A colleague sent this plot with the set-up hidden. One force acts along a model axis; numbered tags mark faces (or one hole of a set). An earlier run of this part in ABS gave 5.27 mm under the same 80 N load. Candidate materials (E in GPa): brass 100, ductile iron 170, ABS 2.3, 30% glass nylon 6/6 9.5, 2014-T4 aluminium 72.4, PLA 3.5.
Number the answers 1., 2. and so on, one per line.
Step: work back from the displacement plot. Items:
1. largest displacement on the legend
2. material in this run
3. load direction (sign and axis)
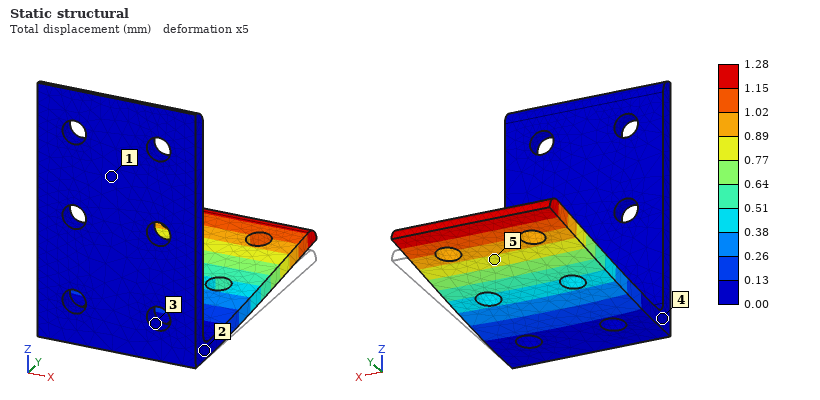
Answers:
1. 1.28 mm
2. 30% glass nylon 6/6
3. +Z
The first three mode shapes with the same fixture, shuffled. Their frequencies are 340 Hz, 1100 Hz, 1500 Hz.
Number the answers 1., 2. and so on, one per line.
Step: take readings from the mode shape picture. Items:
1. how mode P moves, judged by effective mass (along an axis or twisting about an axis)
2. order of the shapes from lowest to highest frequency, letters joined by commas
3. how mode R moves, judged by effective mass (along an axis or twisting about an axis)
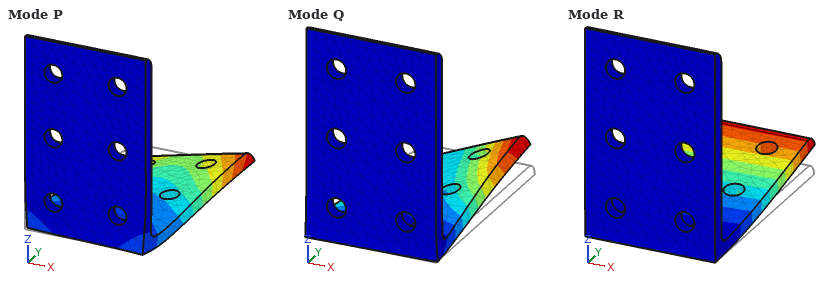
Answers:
1. along X
2. R, Q, P
3. along Z
